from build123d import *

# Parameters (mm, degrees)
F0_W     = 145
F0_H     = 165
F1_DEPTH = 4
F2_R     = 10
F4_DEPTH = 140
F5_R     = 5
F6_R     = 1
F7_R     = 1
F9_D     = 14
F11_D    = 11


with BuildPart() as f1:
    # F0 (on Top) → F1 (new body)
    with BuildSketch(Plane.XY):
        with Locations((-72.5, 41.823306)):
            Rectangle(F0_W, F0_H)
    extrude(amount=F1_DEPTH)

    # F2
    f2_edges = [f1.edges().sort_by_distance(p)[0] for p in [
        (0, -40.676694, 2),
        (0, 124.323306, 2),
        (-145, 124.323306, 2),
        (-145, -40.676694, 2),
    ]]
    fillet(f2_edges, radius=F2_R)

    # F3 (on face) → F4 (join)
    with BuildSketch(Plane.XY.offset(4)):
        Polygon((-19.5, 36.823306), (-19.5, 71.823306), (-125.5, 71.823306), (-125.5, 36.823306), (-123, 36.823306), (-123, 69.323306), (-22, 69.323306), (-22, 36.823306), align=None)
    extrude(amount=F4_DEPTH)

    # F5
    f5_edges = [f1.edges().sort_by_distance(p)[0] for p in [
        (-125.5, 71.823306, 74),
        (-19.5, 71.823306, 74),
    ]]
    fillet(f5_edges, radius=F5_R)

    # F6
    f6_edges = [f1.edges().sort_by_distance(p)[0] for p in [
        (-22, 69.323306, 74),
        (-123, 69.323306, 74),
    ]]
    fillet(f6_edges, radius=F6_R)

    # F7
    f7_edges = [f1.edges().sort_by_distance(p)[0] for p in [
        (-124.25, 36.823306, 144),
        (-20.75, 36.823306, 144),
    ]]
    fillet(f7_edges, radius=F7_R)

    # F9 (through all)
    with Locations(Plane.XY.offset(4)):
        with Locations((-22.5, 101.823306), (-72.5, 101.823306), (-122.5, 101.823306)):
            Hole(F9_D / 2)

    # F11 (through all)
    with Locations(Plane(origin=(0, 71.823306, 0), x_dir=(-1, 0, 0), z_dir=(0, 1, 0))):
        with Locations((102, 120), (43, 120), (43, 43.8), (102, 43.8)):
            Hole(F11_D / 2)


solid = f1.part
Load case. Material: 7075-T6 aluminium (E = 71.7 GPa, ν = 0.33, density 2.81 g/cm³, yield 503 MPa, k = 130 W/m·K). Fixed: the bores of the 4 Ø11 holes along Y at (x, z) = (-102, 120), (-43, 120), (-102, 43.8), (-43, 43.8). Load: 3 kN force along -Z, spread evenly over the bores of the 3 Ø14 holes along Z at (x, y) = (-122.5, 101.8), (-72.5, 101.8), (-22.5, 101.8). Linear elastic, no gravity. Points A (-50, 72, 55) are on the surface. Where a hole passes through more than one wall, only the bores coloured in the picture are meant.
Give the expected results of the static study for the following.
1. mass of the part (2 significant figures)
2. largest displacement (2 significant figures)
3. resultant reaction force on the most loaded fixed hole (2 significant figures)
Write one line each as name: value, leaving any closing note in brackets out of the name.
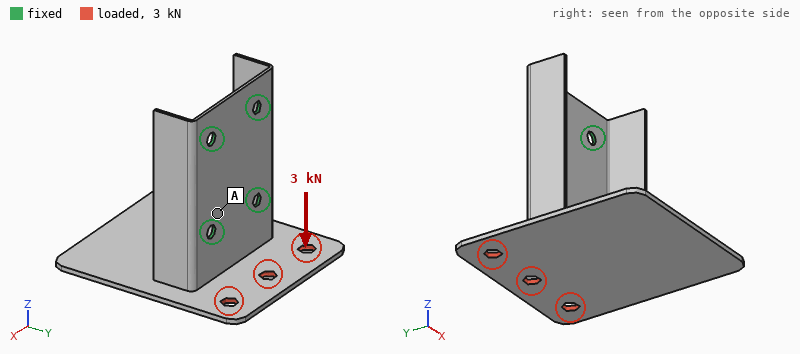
mass of the part: 420 g
largest displacement: 2.2 mm
resultant reaction force on the most loaded fixed hole: 2.1 kN
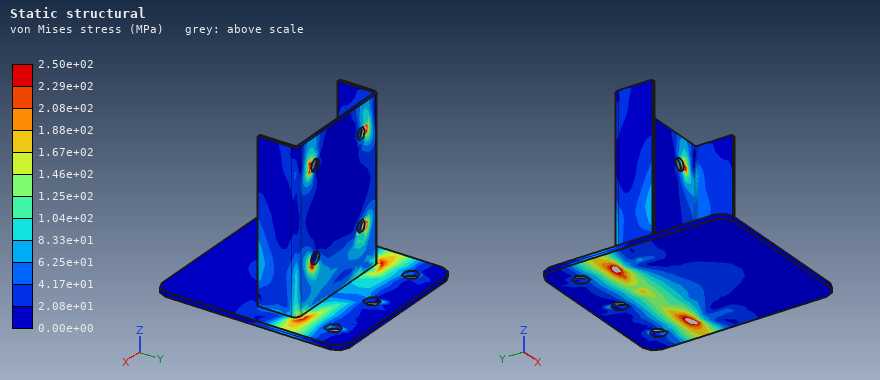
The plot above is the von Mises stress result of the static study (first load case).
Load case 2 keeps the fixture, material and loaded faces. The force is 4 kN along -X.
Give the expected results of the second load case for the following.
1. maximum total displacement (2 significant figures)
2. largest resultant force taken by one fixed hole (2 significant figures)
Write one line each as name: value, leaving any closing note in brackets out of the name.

maximum total displacement: 2.5 mm
largest resultant force taken by one fixed hole: 3.1 kN
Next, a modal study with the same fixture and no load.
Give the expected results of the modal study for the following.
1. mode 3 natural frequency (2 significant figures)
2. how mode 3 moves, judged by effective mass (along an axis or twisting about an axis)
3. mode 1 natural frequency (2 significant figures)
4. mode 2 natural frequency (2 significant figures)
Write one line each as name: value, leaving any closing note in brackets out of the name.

mode 3 natural frequency: 580 Hz
how mode 3 moves, judged by effective mass: along Y
mode 1 natural frequency: 340 Hz
mode 2 natural frequency: 340 Hz
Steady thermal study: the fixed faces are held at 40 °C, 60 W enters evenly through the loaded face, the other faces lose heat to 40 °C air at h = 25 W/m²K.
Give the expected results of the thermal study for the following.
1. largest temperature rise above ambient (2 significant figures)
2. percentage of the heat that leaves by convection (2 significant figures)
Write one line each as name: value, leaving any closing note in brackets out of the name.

largest temperature rise above ambient: 52 K
percentage of the heat that leaves by convection: 62 %
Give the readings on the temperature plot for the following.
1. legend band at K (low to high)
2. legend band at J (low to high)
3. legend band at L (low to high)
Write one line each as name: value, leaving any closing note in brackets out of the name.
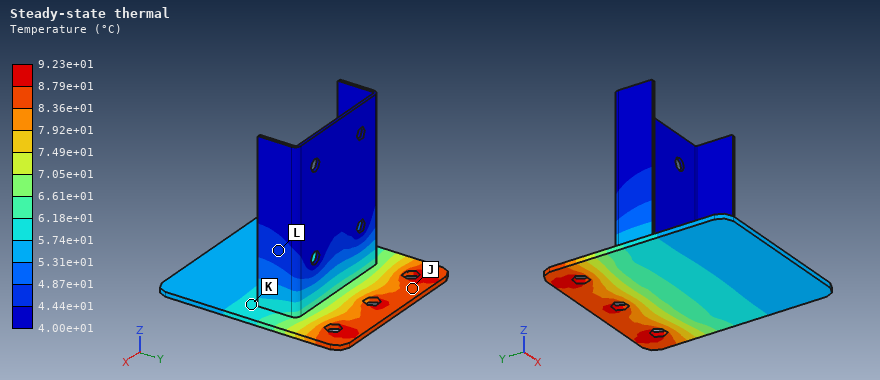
legend band at K: 5.74e+01 to 6.18e+01 °C
legend band at J: 8.36e+01 to 8.79e+01 °C
legend band at L: 4.44e+01 to 4.87e+01 °C
